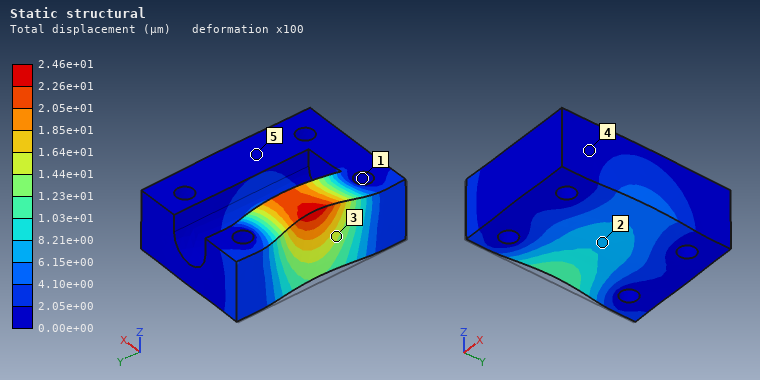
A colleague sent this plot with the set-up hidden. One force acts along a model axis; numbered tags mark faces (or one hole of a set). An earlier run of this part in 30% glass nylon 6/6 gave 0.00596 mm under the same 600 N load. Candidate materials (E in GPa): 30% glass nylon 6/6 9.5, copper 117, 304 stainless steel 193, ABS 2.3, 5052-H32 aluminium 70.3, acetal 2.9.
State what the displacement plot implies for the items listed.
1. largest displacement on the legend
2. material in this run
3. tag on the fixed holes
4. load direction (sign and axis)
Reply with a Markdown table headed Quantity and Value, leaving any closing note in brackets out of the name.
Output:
| Quantity | Value |
|---|---|
| largest displacement on the legend | 2.46e+01 µm |
| material in this run | ABS |
| tag on the fixed holes | 1 |
| load direction | +X |
